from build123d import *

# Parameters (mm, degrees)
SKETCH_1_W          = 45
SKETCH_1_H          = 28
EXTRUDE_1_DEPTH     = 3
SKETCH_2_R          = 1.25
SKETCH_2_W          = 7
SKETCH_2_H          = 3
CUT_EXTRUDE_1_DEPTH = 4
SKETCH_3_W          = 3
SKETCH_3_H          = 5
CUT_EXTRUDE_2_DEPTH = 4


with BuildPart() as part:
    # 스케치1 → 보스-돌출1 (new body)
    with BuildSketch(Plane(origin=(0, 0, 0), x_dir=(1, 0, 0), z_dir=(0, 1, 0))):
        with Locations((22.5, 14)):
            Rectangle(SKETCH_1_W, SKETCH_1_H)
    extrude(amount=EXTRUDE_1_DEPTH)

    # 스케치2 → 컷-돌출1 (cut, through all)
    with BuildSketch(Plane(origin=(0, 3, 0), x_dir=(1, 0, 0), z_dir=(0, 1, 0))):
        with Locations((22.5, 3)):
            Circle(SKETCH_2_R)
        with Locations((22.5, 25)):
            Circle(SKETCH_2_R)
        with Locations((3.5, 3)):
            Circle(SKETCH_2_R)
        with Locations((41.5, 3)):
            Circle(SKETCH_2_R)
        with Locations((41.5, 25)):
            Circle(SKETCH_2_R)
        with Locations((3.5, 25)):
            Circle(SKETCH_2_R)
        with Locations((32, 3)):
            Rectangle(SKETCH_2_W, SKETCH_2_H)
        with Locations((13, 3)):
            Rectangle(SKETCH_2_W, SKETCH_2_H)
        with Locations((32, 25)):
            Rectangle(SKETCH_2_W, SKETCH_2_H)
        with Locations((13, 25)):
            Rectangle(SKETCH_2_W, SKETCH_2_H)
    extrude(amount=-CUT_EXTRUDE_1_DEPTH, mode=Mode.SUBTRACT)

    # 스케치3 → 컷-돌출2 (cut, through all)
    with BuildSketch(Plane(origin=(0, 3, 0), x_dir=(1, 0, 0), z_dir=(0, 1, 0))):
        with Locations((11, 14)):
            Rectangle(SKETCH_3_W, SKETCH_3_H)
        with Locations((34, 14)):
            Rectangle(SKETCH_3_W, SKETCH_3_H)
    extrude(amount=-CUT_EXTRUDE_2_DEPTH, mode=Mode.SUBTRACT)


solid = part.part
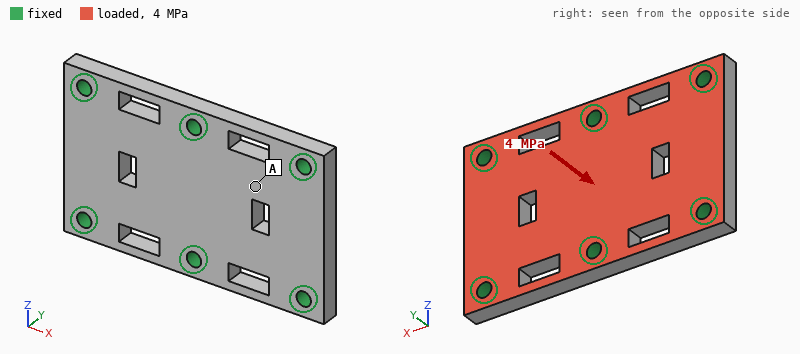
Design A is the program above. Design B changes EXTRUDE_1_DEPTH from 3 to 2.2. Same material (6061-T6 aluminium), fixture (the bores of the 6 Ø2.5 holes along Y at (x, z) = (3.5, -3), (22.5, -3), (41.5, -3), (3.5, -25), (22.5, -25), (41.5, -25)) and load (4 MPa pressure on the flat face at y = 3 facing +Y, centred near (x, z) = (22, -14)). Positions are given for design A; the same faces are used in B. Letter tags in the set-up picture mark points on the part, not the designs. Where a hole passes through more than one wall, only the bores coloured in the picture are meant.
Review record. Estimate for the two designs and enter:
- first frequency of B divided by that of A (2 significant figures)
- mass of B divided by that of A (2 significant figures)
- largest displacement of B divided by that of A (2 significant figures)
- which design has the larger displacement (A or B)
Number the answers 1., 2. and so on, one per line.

1. 0.79
2. 0.73
3. 2.2
4. B
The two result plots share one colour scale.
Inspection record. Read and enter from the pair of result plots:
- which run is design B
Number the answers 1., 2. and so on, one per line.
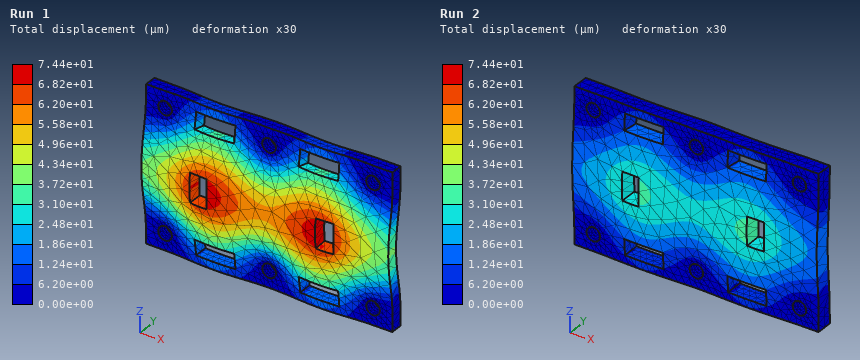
1. Run 1
